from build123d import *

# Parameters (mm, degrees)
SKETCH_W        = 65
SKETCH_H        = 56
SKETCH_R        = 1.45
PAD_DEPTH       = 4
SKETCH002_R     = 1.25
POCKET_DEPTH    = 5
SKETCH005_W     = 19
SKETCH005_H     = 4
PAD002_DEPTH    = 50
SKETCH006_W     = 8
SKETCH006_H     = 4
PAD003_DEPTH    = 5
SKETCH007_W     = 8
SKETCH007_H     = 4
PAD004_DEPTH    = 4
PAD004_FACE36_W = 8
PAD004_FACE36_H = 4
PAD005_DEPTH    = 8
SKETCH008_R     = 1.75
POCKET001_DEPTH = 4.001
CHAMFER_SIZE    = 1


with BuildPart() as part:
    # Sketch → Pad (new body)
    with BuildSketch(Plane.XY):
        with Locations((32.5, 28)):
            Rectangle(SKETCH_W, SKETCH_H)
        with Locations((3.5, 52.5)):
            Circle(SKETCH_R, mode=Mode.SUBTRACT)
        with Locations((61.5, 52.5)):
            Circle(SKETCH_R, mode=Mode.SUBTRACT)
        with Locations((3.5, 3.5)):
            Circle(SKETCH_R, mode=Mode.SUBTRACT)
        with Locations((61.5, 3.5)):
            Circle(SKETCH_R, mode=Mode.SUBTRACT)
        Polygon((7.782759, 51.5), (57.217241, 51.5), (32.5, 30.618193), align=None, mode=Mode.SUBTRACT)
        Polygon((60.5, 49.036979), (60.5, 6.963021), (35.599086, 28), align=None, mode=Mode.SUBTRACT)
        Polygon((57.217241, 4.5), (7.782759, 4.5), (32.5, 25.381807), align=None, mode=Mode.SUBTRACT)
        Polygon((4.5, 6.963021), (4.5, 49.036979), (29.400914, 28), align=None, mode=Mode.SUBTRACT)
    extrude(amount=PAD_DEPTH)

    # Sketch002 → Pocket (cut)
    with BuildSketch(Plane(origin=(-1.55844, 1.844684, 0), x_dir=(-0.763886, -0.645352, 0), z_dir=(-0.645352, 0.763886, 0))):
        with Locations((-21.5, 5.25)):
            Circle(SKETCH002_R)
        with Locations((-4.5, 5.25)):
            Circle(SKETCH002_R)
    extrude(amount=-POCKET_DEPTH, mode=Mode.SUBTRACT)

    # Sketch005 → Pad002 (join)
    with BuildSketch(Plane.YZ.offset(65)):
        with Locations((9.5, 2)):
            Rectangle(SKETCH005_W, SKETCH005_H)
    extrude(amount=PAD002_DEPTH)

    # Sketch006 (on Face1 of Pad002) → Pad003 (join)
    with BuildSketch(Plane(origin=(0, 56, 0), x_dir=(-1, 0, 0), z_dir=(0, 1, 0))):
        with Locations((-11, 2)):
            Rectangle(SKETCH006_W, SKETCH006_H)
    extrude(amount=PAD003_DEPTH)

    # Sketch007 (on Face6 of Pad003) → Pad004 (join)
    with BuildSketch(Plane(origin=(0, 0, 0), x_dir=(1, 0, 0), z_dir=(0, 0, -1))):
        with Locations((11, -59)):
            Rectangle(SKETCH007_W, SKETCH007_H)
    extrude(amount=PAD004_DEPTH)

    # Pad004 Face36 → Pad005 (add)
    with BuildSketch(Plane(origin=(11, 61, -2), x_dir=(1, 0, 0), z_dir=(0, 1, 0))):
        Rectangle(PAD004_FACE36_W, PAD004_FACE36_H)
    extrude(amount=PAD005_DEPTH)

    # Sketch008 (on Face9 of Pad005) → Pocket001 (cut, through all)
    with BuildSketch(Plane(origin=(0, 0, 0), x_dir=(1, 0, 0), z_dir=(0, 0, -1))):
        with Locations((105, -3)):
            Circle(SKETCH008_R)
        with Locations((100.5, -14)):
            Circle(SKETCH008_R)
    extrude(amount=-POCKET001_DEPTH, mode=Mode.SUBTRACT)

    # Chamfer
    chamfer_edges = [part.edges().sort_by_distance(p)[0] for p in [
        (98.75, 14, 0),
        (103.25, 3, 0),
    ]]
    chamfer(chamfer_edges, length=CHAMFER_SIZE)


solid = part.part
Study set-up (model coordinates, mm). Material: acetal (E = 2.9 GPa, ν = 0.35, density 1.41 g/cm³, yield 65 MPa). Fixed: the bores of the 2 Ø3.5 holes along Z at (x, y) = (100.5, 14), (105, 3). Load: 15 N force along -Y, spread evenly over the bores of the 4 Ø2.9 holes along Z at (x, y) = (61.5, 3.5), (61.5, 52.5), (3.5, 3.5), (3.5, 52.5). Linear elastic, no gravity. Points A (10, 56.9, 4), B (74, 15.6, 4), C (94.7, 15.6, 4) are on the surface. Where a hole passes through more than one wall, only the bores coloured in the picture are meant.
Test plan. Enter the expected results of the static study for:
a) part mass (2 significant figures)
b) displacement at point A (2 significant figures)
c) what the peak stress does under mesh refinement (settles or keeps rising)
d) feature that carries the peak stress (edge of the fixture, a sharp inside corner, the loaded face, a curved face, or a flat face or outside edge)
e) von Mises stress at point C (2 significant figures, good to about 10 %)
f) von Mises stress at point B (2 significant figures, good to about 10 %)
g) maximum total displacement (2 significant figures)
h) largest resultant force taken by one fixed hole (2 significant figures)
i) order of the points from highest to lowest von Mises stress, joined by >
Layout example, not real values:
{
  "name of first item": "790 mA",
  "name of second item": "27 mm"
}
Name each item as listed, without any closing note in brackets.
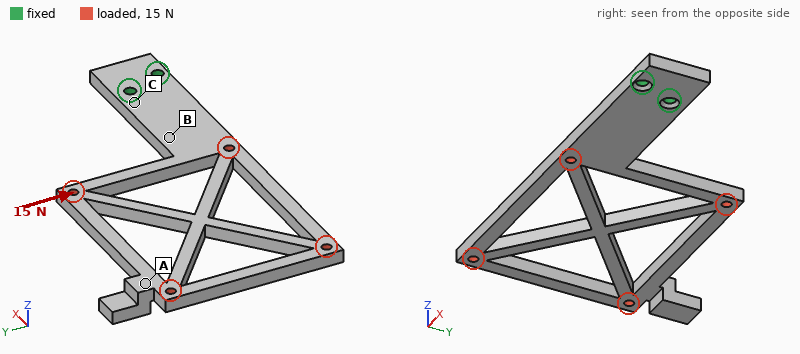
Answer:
{
  "part mass": "15 g",
  "displacement at point A": "1.4 mm",
  "what the peak stress does under mesh refinement": "keeps rising",
  "feature that carries the peak stress": "edge of the fixture",
  "von Mises stress at point C": "2.7 MPa",
  "von Mises stress at point B": "1.6 MPa",
  "maximum total displacement": "1.6 mm",
  "largest resultant force taken by one fixed hole": "80 N",
  "order of the points from highest to lowest von Mises stress, joined by >": "C > B > A"
}
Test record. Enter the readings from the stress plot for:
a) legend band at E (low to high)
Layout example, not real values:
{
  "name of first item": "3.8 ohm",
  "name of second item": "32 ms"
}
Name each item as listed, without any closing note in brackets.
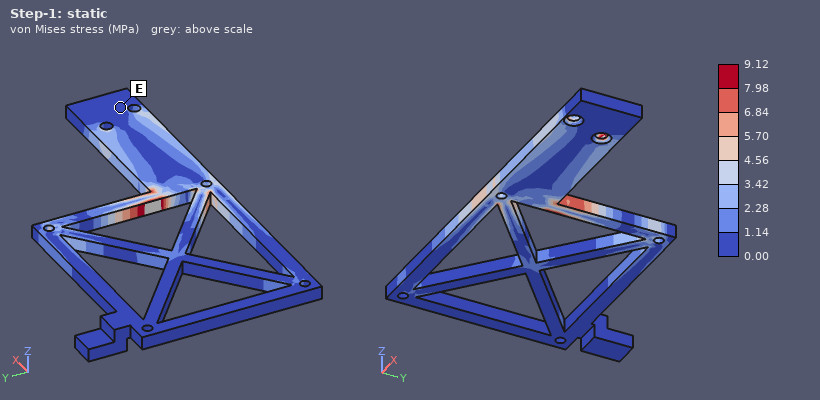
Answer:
{
  "legend band at E": "0.00 to 1.14 MPa"
}
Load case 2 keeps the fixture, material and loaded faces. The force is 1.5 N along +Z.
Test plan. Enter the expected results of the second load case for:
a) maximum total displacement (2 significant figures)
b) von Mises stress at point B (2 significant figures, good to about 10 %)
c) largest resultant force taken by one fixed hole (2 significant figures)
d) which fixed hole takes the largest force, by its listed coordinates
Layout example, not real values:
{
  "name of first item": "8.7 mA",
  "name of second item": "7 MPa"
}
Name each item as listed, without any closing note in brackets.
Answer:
{
  "maximum total displacement": "1.5 mm",
  "von Mises stress at point B": "1.3 MPa",
  "largest resultant force taken by one fixed hole": "5.3 N",
  "which fixed hole takes the largest force, by its listed coordinates": "(100.5, 14)"
}
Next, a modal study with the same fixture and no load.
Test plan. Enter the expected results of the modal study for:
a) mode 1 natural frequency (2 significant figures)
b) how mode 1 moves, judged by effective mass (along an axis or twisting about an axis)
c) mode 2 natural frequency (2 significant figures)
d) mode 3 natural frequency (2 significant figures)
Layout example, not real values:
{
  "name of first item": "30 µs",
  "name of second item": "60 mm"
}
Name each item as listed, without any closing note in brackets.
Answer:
{
  "mode 1 natural frequency": "61 Hz",
  "how mode 1 moves, judged by effective mass": "along Z",
  "mode 2 natural frequency": "160 Hz",
  "mode 3 natural frequency": "170 Hz"
}
